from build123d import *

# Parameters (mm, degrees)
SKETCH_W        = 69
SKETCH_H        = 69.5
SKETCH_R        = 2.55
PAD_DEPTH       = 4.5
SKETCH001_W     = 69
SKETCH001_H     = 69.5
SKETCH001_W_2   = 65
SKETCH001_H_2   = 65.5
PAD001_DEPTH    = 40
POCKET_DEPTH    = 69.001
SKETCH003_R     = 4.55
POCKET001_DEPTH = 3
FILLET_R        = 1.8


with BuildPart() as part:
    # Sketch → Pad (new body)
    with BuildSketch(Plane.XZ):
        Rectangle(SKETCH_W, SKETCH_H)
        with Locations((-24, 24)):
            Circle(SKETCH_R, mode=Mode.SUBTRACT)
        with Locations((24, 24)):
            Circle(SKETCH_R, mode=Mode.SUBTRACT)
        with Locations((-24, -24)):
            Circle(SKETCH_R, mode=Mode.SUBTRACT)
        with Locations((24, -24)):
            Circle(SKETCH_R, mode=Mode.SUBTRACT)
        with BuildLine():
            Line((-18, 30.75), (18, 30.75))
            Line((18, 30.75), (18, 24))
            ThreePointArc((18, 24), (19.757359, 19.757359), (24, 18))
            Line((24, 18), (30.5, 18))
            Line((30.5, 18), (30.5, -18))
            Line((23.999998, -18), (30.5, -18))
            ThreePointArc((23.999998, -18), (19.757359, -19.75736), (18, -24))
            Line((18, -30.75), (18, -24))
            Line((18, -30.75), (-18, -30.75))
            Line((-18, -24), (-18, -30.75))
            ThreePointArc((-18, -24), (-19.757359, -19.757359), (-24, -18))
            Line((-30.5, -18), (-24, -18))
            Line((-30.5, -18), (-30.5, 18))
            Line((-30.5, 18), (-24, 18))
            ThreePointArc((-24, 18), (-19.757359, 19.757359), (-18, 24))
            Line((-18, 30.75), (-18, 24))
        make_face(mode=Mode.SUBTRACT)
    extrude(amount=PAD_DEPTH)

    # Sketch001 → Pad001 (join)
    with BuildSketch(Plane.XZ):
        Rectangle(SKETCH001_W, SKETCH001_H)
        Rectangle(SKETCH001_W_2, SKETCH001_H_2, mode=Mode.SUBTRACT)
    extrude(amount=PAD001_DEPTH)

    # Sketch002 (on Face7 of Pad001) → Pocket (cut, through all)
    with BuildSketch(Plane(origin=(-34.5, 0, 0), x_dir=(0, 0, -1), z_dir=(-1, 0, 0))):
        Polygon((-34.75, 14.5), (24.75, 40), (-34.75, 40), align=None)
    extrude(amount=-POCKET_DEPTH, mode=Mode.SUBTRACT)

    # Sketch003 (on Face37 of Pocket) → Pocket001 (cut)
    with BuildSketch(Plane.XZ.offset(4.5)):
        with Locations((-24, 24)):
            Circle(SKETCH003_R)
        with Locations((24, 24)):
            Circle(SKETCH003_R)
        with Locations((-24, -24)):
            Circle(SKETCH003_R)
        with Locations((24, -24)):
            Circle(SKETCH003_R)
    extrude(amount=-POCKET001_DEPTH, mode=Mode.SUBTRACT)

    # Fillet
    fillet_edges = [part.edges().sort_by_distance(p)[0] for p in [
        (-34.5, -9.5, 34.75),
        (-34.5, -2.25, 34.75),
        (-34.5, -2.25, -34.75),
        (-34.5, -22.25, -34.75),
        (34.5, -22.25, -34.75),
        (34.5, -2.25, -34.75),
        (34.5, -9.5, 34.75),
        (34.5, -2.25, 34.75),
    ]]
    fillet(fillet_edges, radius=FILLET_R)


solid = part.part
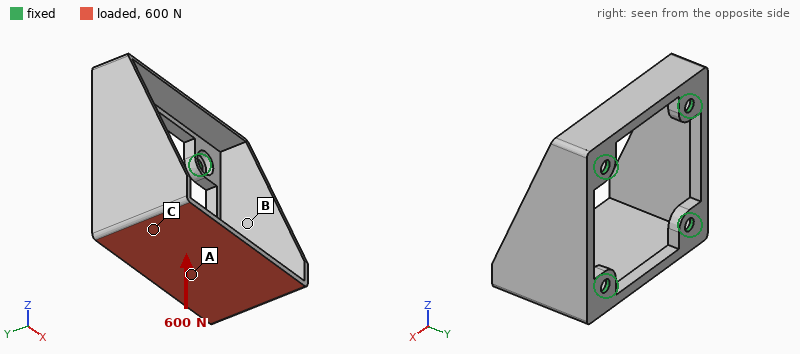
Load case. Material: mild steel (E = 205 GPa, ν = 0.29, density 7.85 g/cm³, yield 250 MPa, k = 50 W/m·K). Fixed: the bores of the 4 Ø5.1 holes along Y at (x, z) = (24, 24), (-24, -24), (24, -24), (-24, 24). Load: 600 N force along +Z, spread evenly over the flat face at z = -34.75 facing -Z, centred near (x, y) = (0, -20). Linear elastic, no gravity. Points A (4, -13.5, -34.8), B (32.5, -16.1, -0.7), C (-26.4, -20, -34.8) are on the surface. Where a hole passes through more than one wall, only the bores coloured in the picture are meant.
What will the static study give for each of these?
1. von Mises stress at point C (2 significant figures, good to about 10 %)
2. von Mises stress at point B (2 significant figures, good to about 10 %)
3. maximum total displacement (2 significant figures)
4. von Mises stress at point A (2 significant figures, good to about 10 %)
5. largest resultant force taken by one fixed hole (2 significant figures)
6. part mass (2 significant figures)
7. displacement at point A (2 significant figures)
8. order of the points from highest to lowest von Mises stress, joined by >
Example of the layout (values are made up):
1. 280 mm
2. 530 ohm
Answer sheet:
1. 44 MPa
2. 8.5 MPa
3. 0.13 mm
4. 29 MPa
5. 310 N
6. 150 g
7. 0.039 mm
8. C > A > B
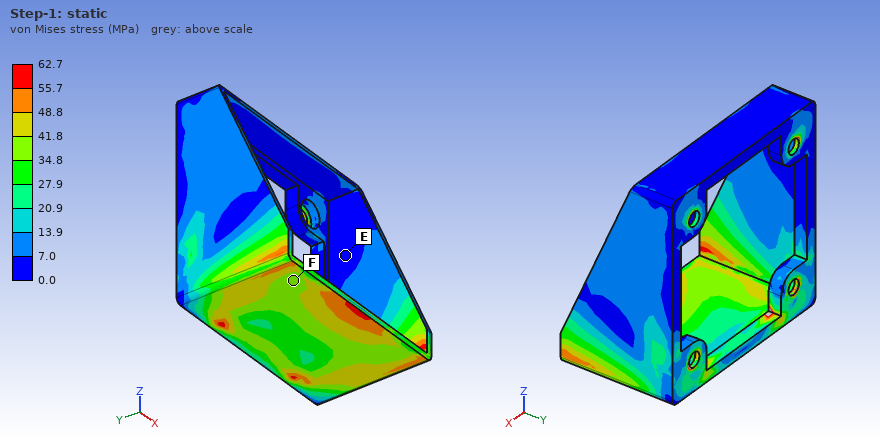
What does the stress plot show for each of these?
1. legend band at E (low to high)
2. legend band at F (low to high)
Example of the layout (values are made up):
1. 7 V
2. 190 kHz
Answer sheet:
1. 0.0 to 7.0 MPa
2. 34.8 to 41.8 MPa
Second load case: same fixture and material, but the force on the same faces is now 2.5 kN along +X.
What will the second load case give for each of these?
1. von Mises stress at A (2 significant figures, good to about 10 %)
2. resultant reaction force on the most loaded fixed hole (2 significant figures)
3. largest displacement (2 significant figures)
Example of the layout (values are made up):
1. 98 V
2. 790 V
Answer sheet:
1. 34 MPa
2. 1.6 kN
3. 48 µm
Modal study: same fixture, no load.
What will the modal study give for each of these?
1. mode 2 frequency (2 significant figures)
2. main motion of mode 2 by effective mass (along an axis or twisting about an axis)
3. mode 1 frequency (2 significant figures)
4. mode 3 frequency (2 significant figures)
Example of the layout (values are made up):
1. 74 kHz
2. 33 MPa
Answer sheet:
1. 2800 Hz
2. along X
3. 2100 Hz
4. 3200 Hz
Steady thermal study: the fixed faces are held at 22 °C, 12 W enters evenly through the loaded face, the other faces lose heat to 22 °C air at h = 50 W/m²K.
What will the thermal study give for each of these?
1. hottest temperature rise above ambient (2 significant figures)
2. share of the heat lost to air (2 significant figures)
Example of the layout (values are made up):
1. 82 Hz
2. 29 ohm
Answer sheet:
1. 28 K
2. 49 %
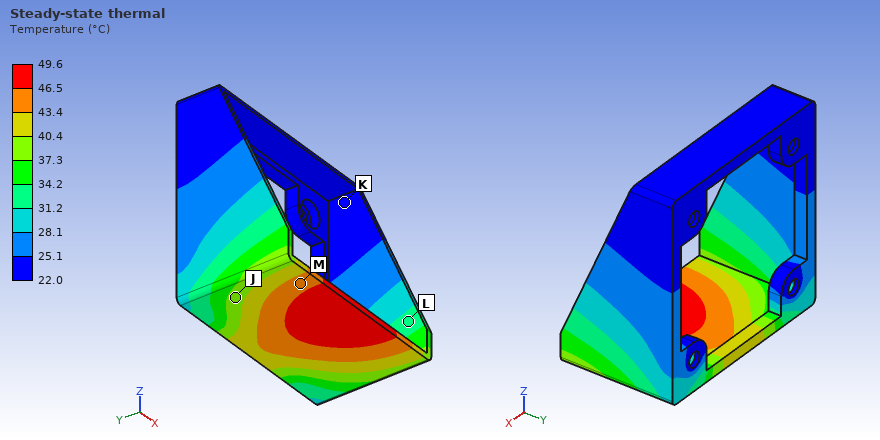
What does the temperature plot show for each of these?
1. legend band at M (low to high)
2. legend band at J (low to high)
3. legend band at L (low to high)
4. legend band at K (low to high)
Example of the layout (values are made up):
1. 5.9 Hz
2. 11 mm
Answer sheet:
1. 43.4 to 46.5 °C
2. 37.3 to 40.4 °C
3. 31.2 to 34.2 °C
4. 22.0 to 25.1 °C
